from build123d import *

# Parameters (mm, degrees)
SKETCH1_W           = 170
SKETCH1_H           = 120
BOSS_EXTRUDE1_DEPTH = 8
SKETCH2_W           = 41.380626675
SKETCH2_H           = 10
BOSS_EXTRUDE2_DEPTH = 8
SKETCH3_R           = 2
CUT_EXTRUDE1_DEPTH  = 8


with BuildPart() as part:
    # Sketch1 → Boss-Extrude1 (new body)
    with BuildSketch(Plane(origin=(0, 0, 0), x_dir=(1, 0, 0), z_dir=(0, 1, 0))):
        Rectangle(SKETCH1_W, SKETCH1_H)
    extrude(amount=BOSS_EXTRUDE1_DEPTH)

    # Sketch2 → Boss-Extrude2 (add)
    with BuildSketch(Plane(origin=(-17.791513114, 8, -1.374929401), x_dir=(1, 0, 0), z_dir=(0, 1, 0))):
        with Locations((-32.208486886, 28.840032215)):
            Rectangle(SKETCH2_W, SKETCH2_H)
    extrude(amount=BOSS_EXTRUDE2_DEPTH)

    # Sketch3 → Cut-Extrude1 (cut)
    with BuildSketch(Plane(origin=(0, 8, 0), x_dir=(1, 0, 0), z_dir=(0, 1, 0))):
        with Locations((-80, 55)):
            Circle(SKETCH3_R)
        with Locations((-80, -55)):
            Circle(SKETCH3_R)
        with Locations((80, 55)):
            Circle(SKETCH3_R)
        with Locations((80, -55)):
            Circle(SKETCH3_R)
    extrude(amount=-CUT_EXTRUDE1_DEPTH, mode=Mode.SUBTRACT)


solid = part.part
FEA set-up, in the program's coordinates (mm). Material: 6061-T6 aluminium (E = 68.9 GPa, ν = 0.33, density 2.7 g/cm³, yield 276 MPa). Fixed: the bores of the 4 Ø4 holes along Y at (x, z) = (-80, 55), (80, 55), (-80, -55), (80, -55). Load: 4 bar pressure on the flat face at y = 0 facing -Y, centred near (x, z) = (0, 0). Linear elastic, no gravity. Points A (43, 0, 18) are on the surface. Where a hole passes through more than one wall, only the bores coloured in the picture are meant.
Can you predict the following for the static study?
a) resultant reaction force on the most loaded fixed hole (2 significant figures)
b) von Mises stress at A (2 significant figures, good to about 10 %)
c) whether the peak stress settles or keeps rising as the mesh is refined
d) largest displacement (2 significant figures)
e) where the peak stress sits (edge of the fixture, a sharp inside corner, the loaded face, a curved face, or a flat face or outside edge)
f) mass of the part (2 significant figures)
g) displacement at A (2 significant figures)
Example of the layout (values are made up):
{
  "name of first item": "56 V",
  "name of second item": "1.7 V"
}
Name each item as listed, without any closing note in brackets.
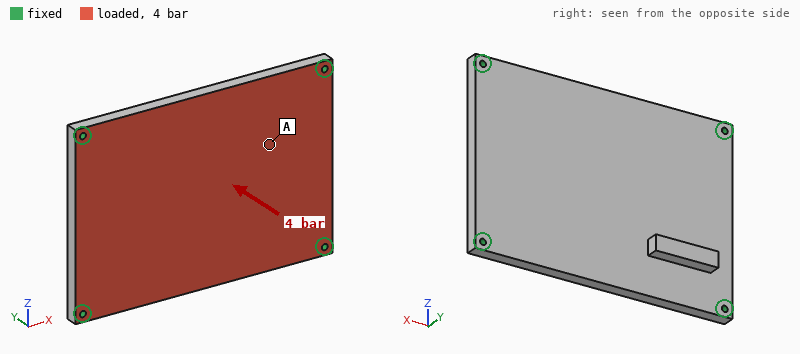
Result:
{
  "resultant reaction force on the most loaded fixed hole": "2.0 kN",
  "von Mises stress at A": "31 MPa",
  "whether the peak stress settles or keeps rising as the mesh is refined": "keeps rising",
  "largest displacement": "0.50 mm",
  "where the peak stress sits": "edge of the fixture",
  "mass of the part": "450 g",
  "displacement at A": "0.34 mm"
}
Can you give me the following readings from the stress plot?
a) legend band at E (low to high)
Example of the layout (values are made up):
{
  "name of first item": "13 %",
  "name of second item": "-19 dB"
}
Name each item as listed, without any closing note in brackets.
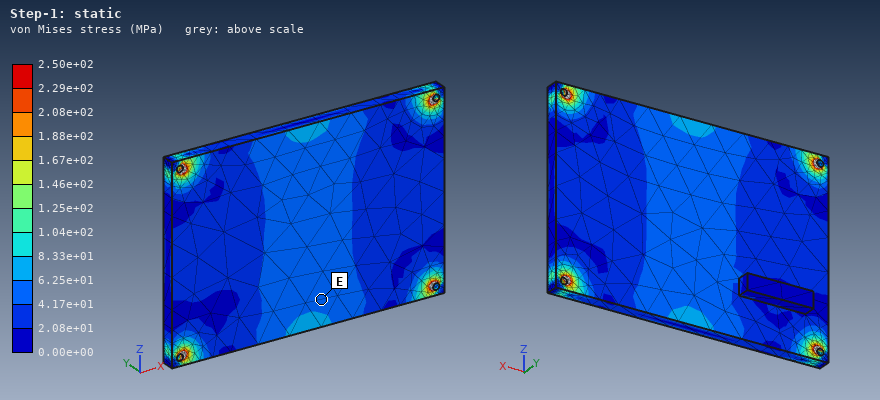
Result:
{
  "legend band at E": "4.17e+01 to 6.25e+01 MPa"
}
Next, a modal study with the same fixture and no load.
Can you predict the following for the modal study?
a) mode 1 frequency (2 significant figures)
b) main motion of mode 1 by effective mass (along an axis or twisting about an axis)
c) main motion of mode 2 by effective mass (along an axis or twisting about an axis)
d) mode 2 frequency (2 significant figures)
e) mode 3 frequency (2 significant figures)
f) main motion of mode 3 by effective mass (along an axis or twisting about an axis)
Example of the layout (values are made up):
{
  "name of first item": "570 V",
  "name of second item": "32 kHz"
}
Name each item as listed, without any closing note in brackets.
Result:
{
  "mode 1 frequency": "1100 Hz",
  "main motion of mode 1 by effective mass": "along Y",
  "main motion of mode 2 by effective mass": "twisting about X",
  "mode 2 frequency": "2000 Hz",
  "mode 3 frequency": "2700 Hz",
  "main motion of mode 3 by effective mass": "twisting about Z"
}
